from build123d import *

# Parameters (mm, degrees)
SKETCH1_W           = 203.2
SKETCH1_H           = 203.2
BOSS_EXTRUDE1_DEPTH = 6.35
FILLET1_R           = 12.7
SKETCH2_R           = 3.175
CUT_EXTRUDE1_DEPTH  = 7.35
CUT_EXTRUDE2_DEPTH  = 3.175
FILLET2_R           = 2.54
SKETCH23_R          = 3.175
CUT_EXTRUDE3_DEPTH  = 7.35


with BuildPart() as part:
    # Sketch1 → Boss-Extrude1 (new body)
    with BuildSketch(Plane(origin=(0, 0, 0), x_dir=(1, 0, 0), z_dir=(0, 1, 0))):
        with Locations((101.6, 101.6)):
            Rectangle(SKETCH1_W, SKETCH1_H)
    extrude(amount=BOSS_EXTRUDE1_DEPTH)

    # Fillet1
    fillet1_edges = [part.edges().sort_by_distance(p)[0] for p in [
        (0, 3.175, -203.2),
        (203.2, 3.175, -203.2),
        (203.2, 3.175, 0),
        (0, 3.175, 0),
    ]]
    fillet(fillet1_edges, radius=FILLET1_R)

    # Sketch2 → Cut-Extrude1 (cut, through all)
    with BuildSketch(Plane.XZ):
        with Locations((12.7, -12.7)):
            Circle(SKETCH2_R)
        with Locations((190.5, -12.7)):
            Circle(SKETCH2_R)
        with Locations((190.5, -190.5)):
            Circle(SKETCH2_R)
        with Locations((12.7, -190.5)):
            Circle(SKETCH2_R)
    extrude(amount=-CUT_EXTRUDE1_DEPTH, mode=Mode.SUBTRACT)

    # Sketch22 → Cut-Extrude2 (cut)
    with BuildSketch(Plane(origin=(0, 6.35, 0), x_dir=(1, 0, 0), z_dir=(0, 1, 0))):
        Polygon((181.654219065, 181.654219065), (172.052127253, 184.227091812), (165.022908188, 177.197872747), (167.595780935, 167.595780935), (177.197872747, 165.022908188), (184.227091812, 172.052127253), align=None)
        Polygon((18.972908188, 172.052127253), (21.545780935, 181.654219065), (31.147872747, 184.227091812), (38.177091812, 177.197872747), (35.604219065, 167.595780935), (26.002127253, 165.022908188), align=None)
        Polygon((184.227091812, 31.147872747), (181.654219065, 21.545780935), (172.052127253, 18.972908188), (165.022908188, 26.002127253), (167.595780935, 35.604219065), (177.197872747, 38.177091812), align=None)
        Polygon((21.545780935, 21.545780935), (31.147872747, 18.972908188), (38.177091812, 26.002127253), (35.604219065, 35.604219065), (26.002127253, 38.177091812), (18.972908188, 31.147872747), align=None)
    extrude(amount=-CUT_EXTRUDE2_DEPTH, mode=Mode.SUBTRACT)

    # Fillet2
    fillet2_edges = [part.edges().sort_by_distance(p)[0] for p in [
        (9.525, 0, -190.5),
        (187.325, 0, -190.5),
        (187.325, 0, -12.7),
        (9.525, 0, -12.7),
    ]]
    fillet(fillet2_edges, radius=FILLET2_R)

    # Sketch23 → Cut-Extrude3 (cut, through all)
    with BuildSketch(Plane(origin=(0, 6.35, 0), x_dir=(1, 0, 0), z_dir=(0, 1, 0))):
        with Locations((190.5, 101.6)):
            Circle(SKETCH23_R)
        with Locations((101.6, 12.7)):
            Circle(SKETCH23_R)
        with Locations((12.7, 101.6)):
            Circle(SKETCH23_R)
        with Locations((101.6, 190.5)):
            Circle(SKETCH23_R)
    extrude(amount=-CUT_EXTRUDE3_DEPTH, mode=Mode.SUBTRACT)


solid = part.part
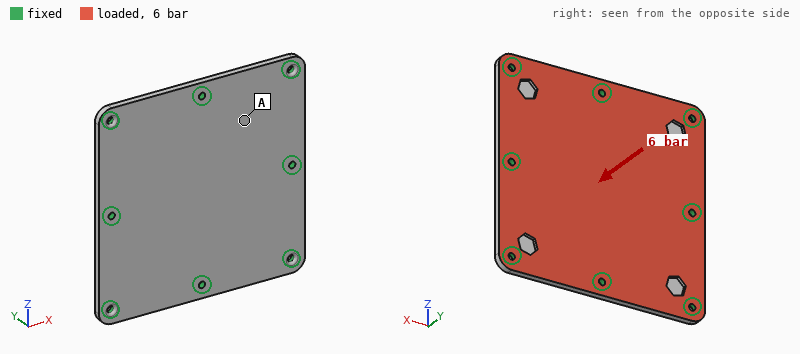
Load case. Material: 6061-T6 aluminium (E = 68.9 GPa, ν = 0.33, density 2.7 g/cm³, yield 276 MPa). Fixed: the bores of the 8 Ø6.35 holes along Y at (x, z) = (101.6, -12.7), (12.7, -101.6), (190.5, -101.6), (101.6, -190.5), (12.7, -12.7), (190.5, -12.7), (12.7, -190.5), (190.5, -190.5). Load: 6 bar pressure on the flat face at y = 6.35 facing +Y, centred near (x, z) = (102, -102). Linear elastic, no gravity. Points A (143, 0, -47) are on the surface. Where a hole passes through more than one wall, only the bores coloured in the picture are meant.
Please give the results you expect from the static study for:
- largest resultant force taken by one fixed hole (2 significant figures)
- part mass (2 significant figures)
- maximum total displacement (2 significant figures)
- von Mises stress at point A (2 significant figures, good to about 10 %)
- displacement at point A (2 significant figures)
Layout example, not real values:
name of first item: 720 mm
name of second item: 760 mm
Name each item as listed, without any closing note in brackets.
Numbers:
largest resultant force taken by one fixed hole: 4.5 kN
part mass: 690 g
maximum total displacement: 0.67 mm
von Mises stress at point A: 56 MPa
displacement at point A: 0.31 mm
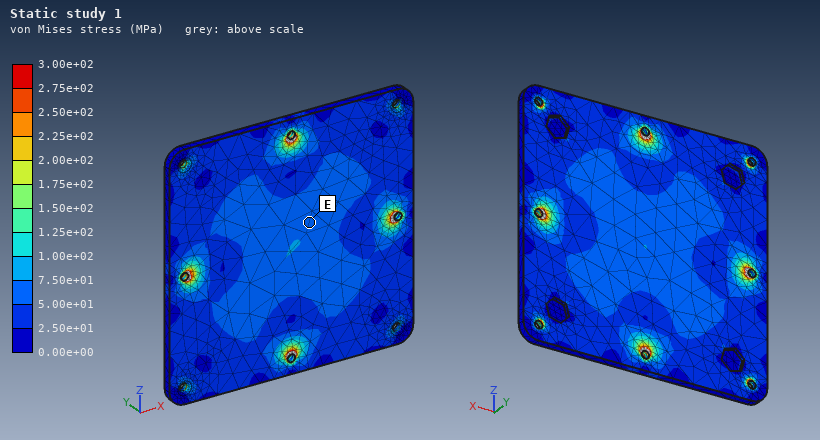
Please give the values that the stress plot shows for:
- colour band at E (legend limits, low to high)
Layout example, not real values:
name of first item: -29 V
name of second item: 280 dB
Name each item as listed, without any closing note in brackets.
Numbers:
colour band at E: 5.00e+01 to 7.50e+01 MPa
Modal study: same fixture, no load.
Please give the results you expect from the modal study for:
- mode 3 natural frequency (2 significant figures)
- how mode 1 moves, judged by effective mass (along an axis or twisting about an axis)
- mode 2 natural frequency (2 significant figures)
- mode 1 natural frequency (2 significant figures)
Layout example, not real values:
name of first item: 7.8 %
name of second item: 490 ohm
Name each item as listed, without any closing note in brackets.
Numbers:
mode 3 natural frequency: 2600 Hz
how mode 1 moves, judged by effective mass: along Y
mode 2 natural frequency: 2600 Hz
mode 1 natural frequency: 1400 Hz
